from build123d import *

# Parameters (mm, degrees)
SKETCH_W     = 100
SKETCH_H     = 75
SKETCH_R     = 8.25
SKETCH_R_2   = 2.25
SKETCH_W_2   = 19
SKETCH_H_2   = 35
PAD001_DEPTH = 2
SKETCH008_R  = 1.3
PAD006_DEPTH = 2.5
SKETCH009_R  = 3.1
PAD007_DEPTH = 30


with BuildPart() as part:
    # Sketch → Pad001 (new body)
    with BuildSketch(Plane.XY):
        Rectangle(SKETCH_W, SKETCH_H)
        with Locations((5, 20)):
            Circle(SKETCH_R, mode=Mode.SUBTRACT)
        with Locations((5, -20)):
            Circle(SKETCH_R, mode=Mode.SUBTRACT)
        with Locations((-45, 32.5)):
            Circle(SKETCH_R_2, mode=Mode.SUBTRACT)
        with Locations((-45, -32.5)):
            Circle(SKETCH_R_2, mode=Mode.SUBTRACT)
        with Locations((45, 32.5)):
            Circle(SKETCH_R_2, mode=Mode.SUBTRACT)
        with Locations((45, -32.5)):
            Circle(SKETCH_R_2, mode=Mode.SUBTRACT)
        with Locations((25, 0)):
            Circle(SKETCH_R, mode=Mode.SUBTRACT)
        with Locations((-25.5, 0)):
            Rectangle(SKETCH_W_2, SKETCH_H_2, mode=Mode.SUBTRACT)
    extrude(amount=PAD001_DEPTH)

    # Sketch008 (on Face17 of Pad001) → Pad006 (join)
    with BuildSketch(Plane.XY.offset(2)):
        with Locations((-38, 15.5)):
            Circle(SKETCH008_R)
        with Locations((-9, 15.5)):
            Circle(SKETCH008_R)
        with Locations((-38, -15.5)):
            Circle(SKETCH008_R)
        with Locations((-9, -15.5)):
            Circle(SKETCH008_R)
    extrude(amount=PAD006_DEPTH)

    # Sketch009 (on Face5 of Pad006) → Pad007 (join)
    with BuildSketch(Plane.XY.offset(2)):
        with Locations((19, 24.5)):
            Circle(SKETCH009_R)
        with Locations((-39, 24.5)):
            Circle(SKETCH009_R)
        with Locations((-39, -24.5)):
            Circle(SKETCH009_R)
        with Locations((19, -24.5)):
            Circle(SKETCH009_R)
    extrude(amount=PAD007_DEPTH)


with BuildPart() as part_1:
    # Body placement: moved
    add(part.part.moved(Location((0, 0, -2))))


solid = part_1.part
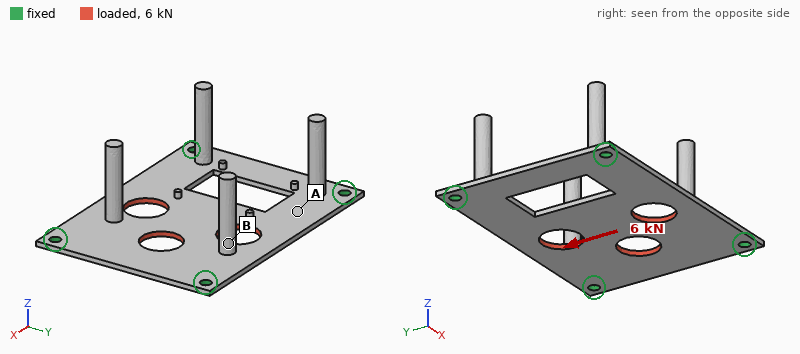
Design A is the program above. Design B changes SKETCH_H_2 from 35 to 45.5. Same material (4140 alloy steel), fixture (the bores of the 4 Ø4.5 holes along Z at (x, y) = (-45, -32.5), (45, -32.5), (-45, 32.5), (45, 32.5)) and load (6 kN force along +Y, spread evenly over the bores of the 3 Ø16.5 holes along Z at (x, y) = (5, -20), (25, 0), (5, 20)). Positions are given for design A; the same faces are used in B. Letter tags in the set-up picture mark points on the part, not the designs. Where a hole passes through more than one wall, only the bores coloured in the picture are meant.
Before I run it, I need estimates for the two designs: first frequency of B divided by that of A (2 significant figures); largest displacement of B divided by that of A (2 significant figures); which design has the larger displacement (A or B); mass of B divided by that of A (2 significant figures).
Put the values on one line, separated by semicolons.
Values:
0.98; 1.1; B; 0.97
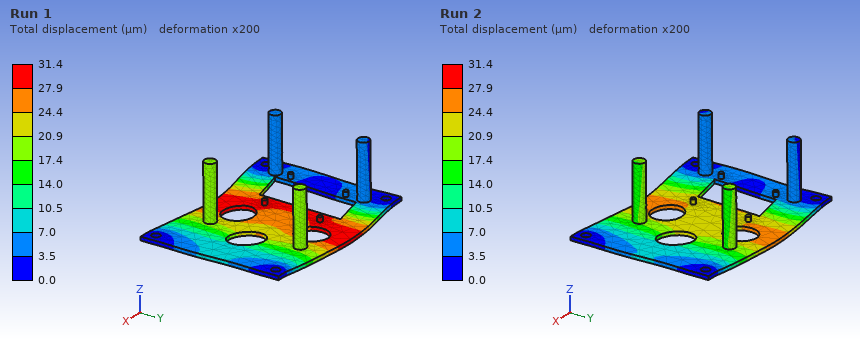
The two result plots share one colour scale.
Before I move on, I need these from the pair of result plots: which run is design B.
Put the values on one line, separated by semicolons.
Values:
Run 1
